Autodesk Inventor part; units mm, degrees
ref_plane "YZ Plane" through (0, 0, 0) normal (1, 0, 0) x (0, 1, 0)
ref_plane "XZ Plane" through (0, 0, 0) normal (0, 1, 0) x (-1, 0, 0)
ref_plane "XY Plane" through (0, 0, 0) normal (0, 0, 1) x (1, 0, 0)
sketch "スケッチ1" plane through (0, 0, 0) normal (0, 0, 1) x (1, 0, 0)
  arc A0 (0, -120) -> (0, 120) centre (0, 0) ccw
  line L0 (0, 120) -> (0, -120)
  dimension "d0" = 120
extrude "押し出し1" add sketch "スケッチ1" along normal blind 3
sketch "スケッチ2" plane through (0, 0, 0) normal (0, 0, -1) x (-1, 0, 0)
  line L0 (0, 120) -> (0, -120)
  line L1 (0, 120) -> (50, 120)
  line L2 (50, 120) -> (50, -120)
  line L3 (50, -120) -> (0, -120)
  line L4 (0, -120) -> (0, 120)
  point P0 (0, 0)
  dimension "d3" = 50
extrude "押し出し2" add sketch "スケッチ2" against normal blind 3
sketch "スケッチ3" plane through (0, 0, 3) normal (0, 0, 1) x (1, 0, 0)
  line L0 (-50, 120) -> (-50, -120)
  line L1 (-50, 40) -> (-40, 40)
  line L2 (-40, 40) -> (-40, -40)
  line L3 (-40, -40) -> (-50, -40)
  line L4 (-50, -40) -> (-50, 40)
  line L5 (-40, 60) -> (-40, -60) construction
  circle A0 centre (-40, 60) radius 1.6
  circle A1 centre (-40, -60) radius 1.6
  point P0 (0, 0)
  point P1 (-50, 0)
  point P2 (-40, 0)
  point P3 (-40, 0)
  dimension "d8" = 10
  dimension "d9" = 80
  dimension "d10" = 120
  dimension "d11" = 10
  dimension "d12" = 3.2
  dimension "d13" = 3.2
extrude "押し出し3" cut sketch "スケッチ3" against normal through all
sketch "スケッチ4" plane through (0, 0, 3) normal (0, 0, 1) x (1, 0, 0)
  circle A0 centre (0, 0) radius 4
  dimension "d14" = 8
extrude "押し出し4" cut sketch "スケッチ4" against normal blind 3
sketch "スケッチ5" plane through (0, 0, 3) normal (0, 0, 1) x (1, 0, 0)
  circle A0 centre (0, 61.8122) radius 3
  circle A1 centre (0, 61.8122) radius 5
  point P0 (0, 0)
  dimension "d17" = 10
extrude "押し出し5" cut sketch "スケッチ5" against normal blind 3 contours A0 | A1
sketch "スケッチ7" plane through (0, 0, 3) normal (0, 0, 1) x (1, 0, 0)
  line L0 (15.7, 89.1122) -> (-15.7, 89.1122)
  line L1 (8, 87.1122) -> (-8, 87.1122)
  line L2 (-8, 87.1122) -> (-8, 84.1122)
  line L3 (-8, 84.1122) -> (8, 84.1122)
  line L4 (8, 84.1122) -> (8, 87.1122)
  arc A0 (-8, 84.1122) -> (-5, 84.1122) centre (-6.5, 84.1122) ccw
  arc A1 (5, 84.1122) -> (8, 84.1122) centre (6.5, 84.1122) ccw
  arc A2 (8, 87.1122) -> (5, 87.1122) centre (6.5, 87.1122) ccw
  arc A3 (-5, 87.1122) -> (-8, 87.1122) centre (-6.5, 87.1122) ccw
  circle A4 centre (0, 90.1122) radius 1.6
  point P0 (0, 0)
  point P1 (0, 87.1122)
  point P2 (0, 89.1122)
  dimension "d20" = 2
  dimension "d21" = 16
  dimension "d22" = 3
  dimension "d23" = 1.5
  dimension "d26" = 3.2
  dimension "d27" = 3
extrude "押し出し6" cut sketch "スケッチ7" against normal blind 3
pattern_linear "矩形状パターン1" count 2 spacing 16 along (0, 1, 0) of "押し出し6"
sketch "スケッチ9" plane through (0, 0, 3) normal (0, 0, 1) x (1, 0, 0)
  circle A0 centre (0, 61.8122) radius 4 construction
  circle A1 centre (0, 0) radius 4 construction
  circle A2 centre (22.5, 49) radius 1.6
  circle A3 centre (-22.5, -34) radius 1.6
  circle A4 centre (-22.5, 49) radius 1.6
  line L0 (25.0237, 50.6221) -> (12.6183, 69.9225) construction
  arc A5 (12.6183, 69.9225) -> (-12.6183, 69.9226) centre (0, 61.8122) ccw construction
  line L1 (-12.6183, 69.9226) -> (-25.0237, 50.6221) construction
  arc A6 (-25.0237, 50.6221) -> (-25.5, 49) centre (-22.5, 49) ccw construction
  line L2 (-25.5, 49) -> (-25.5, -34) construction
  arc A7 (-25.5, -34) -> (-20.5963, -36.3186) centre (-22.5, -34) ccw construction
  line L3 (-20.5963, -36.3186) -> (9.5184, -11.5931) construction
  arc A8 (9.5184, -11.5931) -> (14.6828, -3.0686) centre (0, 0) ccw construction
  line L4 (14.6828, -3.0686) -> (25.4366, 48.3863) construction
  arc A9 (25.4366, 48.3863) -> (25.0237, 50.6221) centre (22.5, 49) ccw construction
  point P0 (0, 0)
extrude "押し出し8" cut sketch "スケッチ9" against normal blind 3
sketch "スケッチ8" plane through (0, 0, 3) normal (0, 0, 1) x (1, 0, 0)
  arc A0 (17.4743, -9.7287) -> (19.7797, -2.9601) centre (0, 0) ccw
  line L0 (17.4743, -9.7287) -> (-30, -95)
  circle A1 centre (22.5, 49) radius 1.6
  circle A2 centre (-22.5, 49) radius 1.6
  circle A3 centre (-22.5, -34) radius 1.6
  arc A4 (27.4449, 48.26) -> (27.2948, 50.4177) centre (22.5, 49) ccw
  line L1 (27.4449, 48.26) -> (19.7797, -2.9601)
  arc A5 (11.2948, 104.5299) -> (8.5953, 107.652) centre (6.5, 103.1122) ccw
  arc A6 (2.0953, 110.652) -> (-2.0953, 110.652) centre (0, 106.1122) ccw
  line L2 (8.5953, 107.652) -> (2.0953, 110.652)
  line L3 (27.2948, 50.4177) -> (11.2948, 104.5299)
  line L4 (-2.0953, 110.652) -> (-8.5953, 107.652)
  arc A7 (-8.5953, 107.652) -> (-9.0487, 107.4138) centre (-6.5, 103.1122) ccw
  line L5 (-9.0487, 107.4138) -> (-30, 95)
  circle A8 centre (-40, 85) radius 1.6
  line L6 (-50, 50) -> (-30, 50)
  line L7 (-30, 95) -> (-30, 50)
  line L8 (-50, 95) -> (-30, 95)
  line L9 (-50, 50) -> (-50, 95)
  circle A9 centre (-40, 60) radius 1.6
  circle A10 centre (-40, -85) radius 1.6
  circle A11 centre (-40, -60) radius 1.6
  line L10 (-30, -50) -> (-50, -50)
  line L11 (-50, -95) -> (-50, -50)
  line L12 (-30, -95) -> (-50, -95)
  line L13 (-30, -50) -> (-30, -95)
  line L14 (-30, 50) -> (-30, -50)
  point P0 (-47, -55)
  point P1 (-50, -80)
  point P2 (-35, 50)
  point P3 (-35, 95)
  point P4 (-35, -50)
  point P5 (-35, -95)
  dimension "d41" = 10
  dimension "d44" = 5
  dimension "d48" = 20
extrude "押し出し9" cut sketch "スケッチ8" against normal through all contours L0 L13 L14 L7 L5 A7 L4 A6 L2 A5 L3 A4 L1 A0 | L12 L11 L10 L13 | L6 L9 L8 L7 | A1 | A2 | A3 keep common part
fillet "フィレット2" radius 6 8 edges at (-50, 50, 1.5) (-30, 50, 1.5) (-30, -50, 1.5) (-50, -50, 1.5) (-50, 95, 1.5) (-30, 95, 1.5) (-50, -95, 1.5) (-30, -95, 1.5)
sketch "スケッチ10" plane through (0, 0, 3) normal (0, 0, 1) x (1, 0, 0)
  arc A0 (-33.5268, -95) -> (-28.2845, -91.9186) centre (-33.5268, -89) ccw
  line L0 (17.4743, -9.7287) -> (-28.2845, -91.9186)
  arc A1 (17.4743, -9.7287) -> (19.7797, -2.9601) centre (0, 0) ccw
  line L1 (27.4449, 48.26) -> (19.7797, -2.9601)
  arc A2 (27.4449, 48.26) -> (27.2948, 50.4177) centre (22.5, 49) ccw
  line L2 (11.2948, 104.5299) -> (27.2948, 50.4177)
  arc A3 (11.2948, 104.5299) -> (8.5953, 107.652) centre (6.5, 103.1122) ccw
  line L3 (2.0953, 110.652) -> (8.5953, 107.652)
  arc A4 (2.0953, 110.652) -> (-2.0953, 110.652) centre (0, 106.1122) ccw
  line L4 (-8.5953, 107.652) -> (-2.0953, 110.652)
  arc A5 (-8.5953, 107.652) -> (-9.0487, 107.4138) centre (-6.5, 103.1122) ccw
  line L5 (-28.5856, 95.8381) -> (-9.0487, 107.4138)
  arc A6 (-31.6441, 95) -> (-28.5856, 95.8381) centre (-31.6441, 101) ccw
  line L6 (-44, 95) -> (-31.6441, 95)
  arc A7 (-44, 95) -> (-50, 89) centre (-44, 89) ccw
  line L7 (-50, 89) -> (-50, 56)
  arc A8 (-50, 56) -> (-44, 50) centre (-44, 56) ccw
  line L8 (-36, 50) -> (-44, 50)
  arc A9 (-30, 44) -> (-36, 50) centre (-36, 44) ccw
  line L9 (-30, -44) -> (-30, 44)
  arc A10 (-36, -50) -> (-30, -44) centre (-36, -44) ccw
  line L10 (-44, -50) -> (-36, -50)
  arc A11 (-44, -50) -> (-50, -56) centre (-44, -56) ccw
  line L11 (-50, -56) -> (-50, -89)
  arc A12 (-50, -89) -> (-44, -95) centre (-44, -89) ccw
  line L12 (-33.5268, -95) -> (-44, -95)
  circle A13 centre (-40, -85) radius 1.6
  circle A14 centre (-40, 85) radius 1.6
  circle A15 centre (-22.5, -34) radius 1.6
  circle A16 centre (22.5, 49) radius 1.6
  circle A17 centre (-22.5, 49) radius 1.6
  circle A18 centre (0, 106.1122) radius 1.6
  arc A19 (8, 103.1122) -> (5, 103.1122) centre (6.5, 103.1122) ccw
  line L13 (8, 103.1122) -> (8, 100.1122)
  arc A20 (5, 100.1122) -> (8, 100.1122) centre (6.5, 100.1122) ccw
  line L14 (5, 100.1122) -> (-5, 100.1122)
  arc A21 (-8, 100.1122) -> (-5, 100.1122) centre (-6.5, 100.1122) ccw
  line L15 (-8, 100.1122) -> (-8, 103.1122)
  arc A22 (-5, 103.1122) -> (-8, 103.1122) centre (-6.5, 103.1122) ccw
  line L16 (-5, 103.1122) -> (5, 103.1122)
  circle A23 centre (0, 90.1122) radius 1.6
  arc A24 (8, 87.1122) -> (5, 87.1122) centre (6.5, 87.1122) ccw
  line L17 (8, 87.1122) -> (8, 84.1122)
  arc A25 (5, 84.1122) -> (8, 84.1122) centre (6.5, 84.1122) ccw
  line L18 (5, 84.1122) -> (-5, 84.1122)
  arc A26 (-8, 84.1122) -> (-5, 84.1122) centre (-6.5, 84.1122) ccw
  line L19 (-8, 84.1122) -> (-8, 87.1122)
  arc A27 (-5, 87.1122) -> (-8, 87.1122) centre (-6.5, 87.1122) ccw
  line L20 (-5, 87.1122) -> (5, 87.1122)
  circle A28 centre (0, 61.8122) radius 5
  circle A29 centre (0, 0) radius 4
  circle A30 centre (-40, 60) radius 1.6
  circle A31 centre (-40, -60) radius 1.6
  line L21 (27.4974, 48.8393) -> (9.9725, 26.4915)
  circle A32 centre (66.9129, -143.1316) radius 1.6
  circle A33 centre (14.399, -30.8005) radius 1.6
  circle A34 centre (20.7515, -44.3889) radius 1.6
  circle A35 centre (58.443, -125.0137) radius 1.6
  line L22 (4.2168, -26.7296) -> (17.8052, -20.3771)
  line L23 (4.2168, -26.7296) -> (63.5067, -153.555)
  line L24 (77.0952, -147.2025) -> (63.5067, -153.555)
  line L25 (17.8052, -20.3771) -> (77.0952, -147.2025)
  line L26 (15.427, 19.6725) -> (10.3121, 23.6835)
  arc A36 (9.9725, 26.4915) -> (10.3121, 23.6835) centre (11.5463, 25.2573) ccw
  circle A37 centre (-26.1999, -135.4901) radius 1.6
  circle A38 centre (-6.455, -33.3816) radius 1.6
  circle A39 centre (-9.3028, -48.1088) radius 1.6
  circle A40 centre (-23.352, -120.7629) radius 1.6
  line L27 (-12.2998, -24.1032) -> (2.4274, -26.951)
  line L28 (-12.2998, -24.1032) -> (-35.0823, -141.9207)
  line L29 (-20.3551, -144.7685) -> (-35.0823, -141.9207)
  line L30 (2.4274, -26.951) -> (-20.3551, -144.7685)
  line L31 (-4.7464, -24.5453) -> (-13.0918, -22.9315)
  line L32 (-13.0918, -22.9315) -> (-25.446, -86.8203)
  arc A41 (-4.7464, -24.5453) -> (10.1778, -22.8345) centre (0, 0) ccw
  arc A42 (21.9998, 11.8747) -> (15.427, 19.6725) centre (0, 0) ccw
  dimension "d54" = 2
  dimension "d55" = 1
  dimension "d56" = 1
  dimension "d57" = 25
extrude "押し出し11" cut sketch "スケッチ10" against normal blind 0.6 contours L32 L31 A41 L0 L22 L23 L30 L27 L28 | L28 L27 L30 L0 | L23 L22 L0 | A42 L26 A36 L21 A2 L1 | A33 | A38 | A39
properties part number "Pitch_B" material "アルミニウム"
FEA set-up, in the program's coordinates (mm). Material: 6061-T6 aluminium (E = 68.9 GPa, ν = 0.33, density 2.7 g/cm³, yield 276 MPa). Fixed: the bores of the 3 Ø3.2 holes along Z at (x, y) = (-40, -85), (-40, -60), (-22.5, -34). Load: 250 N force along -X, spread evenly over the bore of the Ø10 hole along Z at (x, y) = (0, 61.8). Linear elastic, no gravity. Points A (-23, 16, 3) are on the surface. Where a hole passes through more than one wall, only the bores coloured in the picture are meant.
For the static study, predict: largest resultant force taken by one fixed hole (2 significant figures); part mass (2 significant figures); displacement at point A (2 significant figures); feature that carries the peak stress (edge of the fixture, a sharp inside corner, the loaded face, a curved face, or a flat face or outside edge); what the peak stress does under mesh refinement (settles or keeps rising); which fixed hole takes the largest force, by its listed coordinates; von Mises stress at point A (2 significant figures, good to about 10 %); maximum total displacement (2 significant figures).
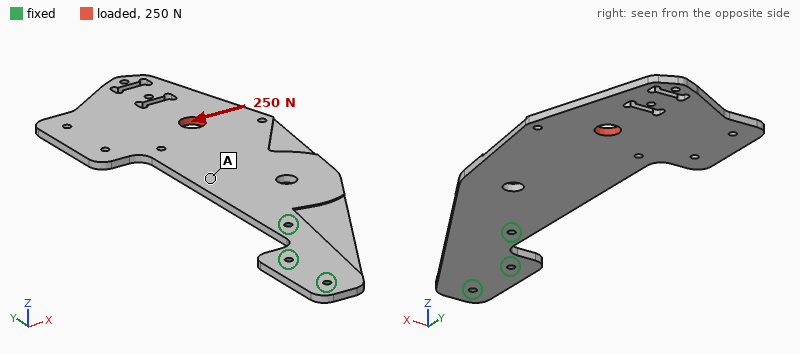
1.1 kN
74 g
0.10 mm
edge of the fixture
keeps rising
(-22.5, -34)
6.3 MPa
0.35 mm
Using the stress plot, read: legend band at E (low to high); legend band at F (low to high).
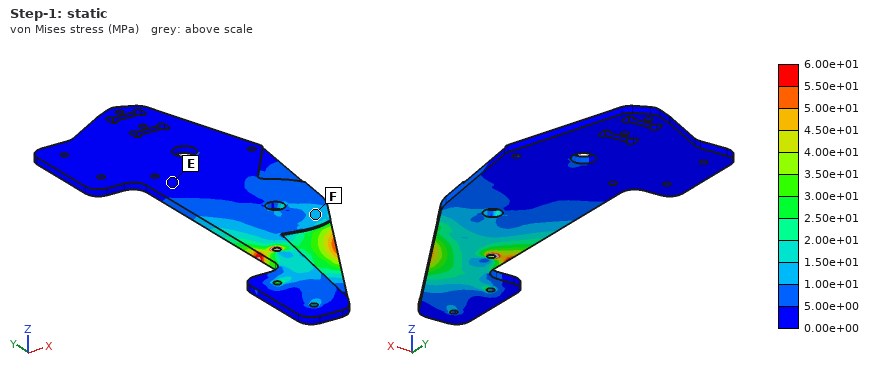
0.00e+00 to 5.00e+00 MPa
1.00e+01 to 1.50e+01 MPa
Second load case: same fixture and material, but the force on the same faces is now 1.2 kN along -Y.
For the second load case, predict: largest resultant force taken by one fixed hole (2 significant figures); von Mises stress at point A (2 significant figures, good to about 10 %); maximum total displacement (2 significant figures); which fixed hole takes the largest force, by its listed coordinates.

1.2 kN
5.9 MPa
0.36 mm
(-22.5, -34)
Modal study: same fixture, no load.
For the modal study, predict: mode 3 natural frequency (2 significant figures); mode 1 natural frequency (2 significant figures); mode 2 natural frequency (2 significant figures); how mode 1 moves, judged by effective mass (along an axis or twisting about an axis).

710 Hz
97 Hz
370 Hz
along Z
